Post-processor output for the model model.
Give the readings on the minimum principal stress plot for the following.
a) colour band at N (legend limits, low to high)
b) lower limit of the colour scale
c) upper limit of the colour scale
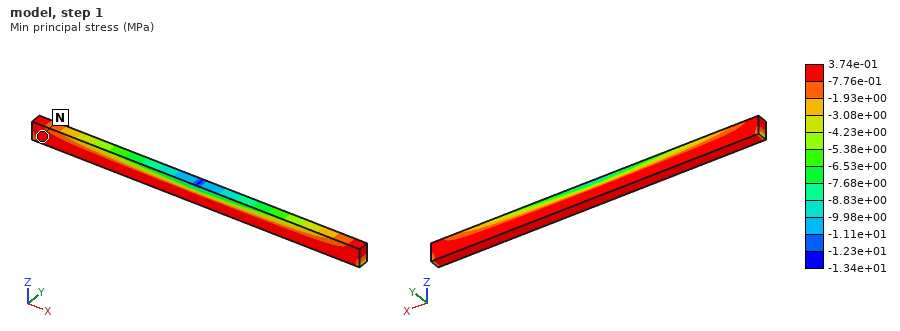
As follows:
-7.76e-01 to 3.74e-01 MPa
-1.34e+01 MPa
3.74e-01 MPa
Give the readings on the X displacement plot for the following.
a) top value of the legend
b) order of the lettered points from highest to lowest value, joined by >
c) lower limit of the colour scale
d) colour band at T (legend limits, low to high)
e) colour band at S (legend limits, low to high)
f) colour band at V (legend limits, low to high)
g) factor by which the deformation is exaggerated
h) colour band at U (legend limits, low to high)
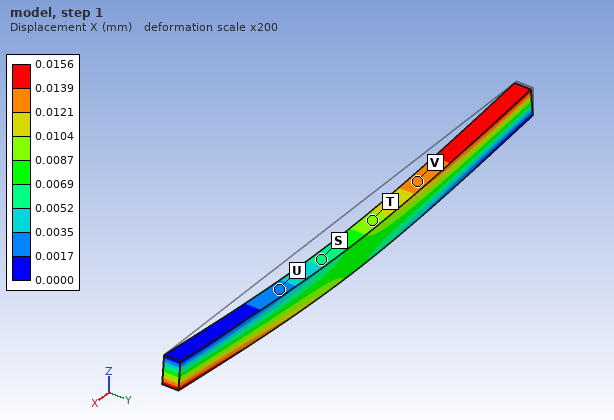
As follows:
0.0156 mm
V > T > S > U
0.0000 mm
0.0087 to 0.0104 mm
0.0052 to 0.0069 mm
0.0121 to 0.0139 mm
200
0.0017 to 0.0035 mm
